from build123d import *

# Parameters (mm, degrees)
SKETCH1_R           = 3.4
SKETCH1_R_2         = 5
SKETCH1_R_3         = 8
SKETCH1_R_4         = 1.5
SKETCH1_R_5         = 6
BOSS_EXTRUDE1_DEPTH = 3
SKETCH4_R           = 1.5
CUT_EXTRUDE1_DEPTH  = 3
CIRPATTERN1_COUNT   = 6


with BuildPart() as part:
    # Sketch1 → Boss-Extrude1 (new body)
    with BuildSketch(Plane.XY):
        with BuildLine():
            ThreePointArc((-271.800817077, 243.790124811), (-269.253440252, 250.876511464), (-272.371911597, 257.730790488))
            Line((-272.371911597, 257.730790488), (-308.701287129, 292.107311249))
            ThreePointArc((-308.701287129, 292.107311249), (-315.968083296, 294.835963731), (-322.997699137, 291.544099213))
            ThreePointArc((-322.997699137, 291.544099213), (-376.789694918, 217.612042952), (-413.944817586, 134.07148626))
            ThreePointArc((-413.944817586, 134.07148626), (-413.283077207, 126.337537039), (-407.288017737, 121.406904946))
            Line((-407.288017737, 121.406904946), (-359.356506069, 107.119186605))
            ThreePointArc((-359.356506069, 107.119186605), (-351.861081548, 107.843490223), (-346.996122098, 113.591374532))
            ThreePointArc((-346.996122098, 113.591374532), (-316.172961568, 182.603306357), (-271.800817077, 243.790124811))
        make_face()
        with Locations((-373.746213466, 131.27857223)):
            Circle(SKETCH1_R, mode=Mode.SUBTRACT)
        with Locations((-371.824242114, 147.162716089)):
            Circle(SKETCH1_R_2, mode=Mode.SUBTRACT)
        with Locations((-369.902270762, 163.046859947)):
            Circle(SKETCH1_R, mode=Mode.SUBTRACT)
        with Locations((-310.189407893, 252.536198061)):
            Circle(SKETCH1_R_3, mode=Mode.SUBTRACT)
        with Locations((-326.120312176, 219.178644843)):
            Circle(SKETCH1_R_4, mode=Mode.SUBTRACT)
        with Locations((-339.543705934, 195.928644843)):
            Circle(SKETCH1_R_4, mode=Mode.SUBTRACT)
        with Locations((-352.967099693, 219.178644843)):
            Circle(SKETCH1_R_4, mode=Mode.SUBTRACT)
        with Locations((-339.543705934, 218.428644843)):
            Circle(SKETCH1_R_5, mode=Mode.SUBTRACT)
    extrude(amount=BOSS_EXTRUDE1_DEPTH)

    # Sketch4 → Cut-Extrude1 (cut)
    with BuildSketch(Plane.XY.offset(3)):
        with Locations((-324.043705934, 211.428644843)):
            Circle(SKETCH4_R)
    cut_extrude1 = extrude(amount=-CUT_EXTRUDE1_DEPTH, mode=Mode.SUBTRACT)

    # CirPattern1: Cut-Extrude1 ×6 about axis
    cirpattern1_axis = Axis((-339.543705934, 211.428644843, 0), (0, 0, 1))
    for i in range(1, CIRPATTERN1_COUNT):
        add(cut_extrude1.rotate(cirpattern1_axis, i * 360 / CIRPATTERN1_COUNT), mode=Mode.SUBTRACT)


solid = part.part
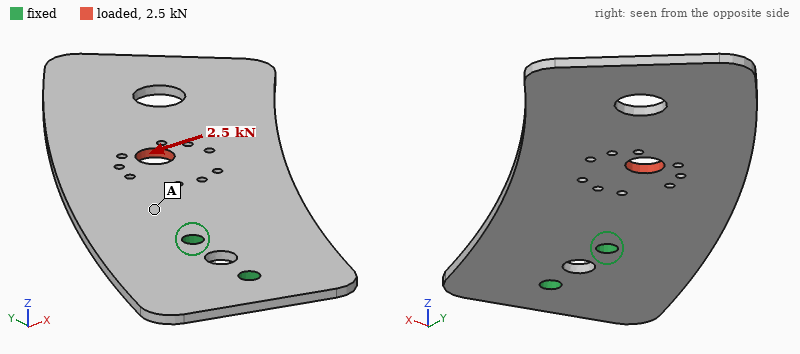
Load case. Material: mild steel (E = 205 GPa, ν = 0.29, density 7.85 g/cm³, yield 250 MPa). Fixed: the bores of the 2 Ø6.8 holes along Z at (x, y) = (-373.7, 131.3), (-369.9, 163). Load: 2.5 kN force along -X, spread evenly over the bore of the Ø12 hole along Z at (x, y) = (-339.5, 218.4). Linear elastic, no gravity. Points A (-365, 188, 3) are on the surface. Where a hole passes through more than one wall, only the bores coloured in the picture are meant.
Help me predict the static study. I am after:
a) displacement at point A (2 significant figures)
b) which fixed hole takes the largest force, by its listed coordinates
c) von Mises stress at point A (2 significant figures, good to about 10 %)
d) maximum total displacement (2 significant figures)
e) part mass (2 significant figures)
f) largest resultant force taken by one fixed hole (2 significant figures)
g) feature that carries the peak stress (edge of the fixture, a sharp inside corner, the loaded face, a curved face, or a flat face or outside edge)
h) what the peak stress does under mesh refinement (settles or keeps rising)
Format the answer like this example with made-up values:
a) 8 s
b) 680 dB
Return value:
a) 0.020 mm
b) (-369.9, 163)
c) 26 MPa
d) 0.11 mm
e) 290 g
f) 6.0 kN
g) edge of the fixture
h) keeps rising
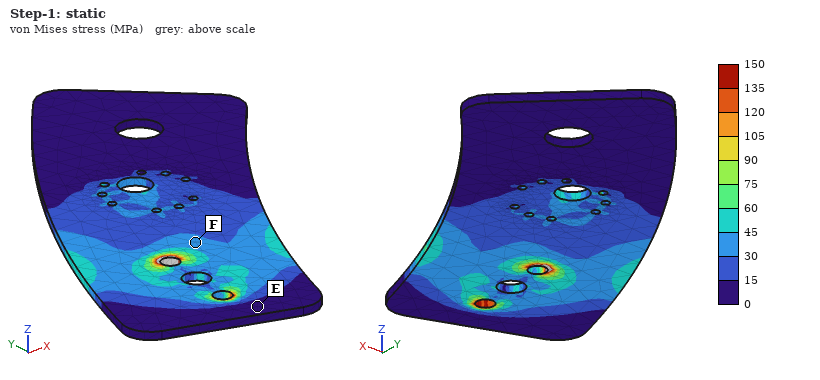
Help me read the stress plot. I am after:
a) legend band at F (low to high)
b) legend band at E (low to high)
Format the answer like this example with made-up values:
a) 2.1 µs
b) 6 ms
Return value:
a) 30 to 45 MPa
b) 0 to 15 MPa
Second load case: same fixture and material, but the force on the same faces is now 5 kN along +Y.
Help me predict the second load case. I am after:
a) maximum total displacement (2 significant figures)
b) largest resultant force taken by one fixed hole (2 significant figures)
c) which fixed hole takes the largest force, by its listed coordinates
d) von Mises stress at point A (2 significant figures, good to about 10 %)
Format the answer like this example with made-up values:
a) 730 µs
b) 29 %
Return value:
a) 0.10 mm
b) 5.5 kN
c) (-369.9, 163)
d) 32 MPa
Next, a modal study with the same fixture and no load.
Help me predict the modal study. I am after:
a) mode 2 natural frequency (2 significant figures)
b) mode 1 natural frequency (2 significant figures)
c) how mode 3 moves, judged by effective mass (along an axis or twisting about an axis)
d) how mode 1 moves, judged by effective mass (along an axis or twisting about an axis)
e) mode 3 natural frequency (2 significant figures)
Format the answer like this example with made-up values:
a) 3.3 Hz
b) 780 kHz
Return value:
a) 480 Hz
b) 130 Hz
c) along Z
d) along Z
e) 770 Hz
